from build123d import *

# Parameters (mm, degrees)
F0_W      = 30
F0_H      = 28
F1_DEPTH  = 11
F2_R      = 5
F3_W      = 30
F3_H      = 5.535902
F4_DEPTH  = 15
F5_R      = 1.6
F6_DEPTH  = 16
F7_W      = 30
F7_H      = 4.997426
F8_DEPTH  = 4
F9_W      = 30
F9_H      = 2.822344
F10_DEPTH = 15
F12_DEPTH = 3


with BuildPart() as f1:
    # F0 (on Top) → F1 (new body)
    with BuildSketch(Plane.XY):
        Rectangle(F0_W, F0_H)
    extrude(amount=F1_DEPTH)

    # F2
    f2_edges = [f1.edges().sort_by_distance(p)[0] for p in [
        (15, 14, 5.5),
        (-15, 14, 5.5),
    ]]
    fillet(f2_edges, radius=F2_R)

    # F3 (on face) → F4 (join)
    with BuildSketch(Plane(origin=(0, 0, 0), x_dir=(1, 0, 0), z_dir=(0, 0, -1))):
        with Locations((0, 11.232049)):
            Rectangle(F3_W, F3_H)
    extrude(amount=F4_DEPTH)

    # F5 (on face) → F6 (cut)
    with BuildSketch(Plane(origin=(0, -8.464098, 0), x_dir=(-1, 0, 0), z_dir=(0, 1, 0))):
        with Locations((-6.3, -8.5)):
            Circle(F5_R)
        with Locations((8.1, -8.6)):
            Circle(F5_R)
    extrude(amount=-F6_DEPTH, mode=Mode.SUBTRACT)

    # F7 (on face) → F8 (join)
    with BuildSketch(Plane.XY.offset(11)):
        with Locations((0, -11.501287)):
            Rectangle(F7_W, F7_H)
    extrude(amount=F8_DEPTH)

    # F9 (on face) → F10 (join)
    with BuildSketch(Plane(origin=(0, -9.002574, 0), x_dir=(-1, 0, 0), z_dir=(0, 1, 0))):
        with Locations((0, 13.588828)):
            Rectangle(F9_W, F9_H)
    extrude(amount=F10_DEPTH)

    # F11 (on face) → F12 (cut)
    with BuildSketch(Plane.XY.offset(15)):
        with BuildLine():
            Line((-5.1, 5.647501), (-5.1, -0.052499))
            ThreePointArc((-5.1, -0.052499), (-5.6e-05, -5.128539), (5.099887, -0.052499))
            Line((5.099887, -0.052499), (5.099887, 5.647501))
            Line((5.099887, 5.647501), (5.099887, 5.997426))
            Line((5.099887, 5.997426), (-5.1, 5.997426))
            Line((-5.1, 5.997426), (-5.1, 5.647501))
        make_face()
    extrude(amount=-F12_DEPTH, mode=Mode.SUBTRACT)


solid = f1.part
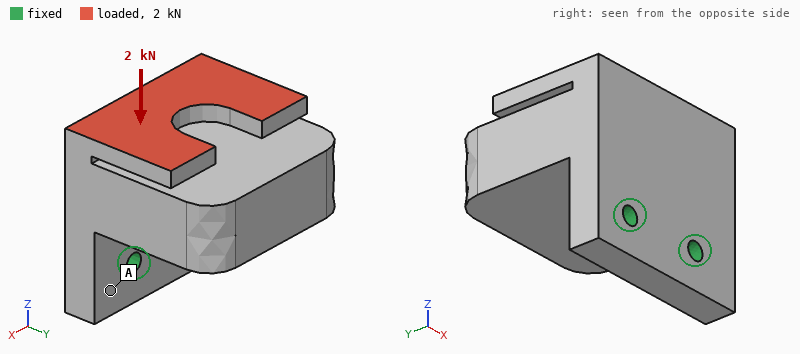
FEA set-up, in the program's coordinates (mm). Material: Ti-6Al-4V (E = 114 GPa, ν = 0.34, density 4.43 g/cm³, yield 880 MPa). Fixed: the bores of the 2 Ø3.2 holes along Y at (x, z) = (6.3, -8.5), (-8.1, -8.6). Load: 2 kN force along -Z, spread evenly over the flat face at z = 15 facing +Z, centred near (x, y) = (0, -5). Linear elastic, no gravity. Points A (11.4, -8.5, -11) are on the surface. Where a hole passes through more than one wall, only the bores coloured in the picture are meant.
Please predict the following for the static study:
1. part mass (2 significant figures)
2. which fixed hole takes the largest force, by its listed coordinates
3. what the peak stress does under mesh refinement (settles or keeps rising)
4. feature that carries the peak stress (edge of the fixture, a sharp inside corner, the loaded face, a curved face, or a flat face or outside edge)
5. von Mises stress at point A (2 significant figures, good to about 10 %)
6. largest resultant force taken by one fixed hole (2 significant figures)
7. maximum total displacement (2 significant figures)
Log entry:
58 g
(6.3, -8.5)
keeps rising
edge of the fixture
24 MPa
1.1 kN
0.22 mm
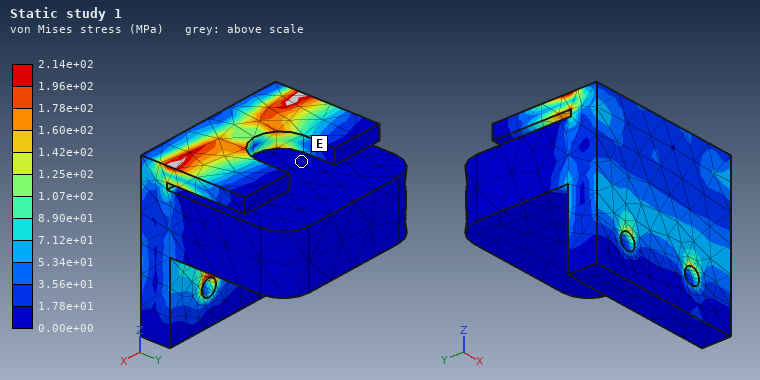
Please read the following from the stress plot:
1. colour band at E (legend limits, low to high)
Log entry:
0.00e+00 to 1.78e+01 MPa
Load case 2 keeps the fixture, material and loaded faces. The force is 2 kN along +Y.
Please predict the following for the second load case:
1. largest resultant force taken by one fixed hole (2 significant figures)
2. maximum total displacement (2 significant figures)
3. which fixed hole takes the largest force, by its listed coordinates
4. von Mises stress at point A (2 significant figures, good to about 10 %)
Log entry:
1.1 kN
0.27 mm
(6.3, -8.5)
67 MPa
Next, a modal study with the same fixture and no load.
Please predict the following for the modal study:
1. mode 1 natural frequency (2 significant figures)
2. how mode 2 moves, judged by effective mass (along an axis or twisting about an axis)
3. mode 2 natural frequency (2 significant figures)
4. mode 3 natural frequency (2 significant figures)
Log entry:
2800 Hz
along X
5600 Hz
9100 Hz
